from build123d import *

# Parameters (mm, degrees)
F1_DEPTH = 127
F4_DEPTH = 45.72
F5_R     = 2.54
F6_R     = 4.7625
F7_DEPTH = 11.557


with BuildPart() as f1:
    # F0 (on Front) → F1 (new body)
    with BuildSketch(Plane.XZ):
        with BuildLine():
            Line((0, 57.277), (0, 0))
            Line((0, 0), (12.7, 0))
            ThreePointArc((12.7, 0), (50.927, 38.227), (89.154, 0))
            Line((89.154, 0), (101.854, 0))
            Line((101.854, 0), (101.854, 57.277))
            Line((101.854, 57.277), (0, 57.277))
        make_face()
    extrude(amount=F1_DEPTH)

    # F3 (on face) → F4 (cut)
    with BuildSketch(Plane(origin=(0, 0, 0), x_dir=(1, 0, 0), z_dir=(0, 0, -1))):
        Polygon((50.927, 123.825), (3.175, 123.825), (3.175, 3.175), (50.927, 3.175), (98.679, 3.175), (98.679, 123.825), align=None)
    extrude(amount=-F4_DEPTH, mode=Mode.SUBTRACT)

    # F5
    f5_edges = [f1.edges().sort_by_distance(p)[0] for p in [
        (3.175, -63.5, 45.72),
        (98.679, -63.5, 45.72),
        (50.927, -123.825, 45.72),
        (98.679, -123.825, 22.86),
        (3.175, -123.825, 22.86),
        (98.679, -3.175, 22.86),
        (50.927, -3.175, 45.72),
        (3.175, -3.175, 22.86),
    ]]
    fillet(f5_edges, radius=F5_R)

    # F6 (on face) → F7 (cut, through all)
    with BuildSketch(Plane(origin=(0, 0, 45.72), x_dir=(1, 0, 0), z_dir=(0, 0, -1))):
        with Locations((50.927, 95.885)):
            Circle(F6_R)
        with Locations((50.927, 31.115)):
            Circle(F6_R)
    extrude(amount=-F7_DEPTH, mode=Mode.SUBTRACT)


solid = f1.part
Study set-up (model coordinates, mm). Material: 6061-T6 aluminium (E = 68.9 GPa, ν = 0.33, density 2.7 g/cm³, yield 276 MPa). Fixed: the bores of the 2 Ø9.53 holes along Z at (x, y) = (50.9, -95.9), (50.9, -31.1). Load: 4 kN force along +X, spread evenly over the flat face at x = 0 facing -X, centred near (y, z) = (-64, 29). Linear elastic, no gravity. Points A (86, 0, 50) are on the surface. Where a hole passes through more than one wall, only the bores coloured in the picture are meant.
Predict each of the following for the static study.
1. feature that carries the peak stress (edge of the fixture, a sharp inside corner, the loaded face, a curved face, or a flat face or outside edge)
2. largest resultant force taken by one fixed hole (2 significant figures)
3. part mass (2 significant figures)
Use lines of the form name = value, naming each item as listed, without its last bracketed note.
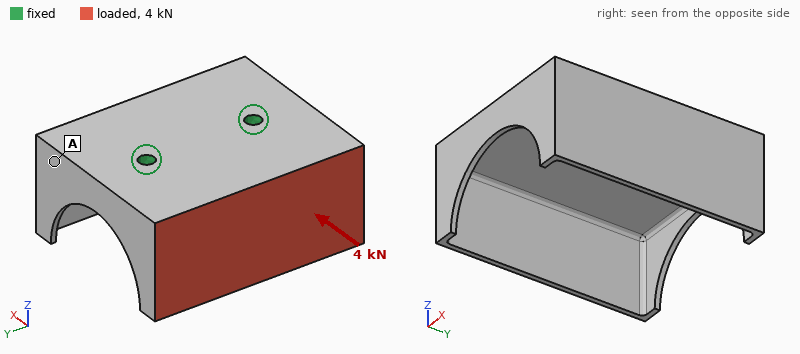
feature that carries the peak stress = a curved face
largest resultant force taken by one fixed hole = 2.1 kN
part mass = 540 g
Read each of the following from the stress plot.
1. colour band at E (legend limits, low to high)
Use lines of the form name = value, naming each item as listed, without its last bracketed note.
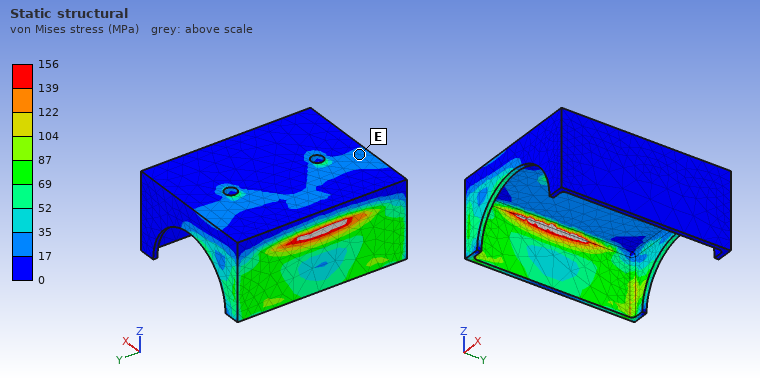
colour band at E = 17 to 35 MPa
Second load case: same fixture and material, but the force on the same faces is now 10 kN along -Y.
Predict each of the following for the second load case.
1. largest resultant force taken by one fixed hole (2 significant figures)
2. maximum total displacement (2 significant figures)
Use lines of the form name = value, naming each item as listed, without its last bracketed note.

largest resultant force taken by one fixed hole = 9.2 kN
maximum total displacement = 0.35 mm
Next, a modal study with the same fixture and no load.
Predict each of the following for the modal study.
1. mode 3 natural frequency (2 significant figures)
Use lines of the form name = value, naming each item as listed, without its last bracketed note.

mode 3 natural frequency = 2100 Hz
